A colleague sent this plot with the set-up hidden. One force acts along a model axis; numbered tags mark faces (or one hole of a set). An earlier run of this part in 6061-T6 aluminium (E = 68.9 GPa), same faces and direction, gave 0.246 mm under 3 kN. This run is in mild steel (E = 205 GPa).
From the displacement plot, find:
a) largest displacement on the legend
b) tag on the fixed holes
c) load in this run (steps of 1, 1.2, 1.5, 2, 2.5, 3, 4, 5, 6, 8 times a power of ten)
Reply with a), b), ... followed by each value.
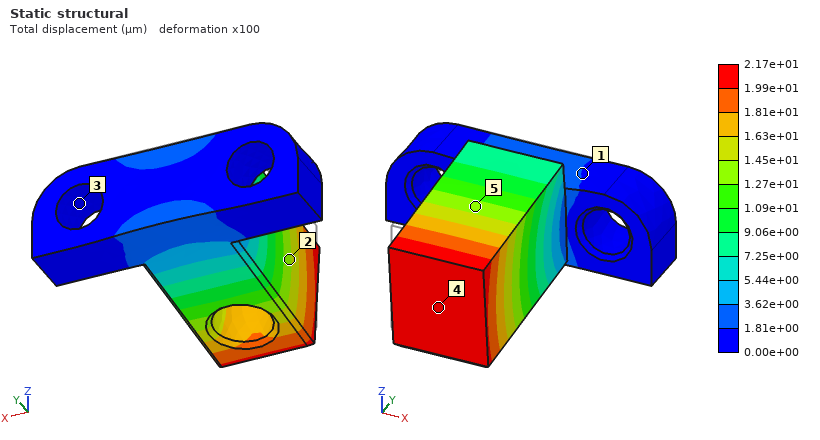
a) 2.17e+01 µm
b) 3
c) 800 N
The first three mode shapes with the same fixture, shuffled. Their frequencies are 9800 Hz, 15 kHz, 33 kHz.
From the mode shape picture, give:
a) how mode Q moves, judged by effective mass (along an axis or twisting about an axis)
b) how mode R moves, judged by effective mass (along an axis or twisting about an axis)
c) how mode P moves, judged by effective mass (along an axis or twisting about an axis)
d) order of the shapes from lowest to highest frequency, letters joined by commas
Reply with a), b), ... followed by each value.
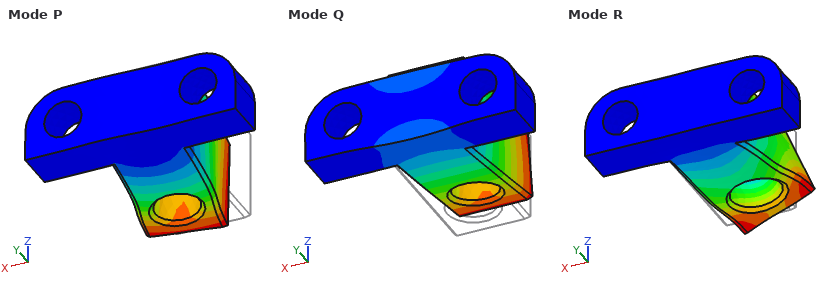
a) along Z
b) twisting about Y
c) along X
d) Q, P, R
